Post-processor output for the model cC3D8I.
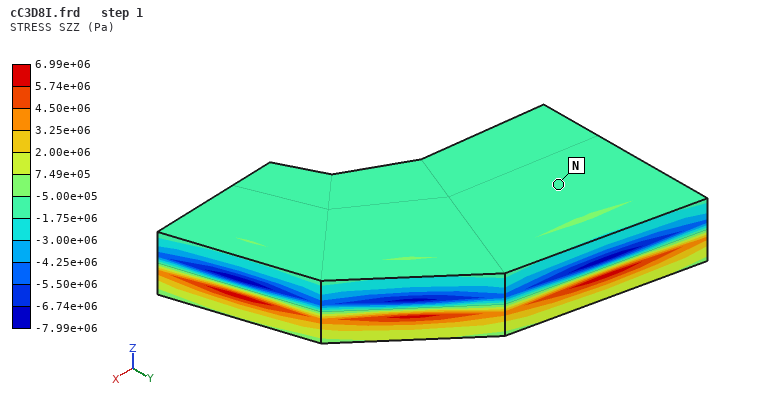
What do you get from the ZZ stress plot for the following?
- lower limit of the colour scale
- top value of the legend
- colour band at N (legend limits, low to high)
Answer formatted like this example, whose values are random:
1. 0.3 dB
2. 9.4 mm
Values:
1. -7.99e+06 Pa
2. 6.99e+06 Pa
3. -1.75e+06 to -5.00e+05 Pa
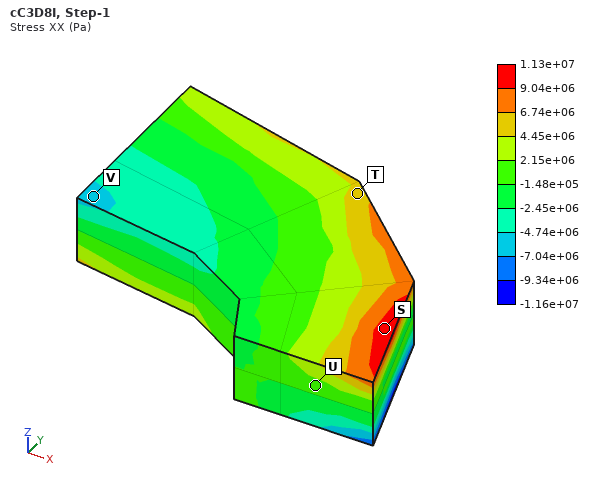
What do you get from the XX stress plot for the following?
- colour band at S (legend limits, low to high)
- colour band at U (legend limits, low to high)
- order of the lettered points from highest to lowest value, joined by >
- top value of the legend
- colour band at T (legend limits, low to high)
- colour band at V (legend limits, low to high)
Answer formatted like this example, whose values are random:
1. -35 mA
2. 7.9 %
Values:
1. 9.04e+06 to 1.13e+07 Pa
2. -1.48e+05 to 2.15e+06 Pa
3. S > T > U > V
4. 1.13e+07 Pa
5. 4.45e+06 to 6.74e+06 Pa
6. -7.04e+06 to -4.74e+06 Pa
